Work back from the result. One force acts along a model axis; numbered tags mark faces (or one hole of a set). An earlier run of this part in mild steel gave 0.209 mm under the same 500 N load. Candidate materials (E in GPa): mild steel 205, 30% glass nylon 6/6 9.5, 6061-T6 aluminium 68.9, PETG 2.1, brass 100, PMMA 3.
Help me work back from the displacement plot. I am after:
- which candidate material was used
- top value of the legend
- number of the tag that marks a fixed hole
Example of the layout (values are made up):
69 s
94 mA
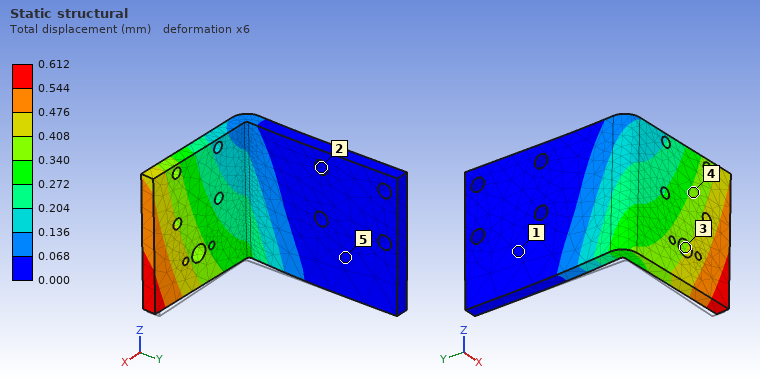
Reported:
6061-T6 aluminium
0.612 mm
2
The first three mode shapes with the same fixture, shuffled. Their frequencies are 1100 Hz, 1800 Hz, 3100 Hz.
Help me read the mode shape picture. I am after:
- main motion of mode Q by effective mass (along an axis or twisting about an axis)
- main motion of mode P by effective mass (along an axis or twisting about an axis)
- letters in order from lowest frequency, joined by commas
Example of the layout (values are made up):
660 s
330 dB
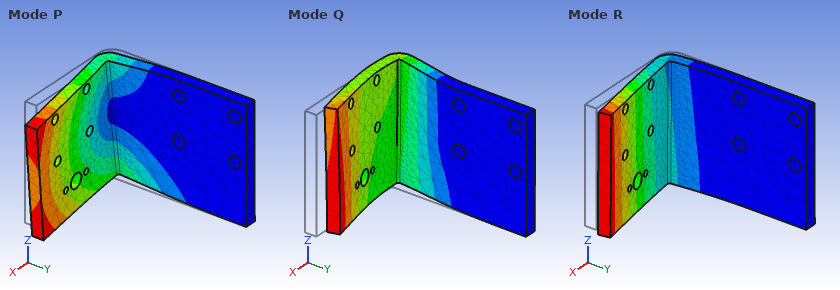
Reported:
along X
along Z
R, P, Q
